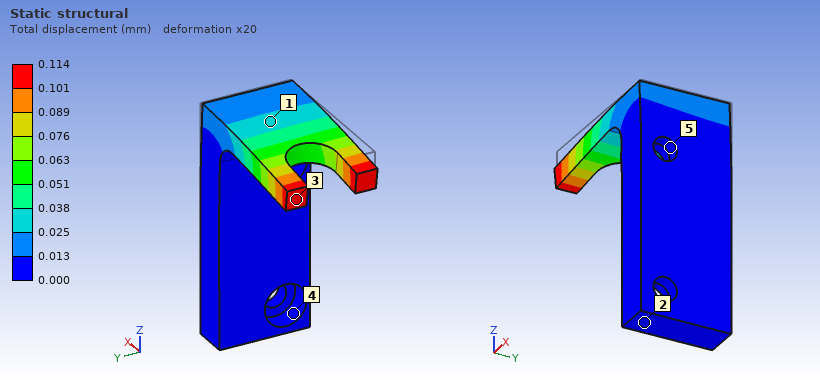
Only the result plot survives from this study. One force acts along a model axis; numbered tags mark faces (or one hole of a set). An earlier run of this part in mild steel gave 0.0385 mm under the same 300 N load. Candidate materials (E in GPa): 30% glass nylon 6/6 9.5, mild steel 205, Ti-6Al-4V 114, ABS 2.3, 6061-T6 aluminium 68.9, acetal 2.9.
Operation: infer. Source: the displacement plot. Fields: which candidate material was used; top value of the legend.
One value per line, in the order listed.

6061-T6 aluminium
0.114 mm
